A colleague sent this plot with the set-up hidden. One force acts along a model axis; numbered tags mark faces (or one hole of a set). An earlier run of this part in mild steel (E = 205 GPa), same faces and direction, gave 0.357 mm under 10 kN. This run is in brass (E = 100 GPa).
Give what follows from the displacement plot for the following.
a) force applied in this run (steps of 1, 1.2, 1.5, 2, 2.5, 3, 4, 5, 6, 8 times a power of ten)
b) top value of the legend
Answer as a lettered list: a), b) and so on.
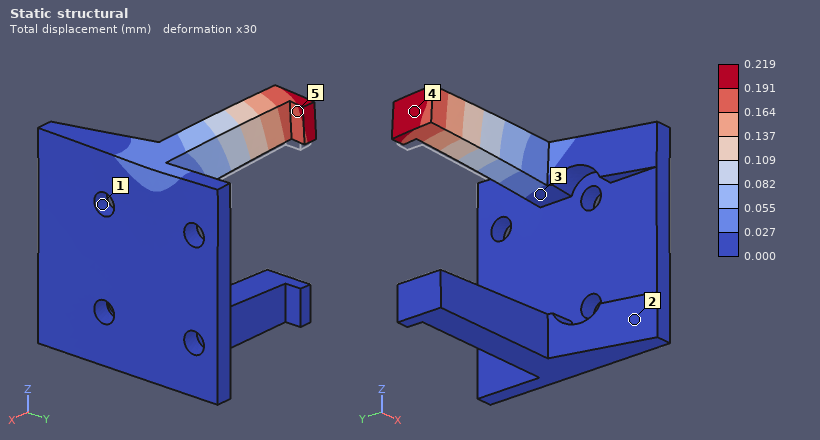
a) 3 kN
b) 0.219 mm
